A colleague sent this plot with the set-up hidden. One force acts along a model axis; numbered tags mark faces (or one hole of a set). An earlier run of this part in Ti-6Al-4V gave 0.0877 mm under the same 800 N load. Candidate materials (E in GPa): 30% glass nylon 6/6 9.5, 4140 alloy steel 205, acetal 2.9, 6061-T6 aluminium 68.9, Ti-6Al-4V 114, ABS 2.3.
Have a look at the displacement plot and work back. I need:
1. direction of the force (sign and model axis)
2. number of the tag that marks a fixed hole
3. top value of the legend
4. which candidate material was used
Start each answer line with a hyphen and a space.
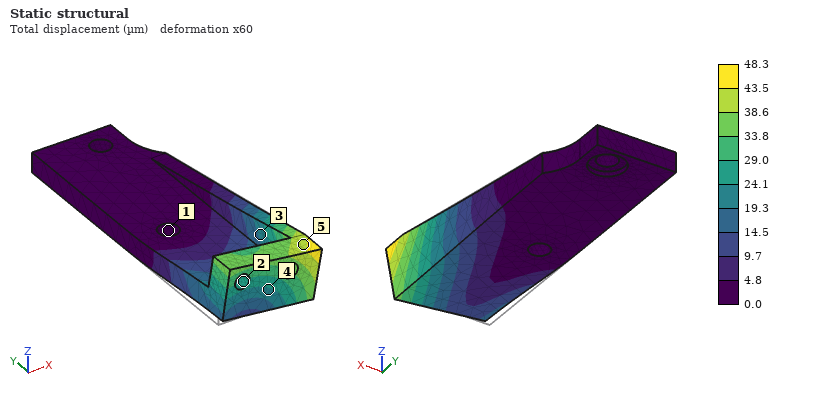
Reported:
- +X
- 1
- 48.3 µm
- 4140 alloy steel
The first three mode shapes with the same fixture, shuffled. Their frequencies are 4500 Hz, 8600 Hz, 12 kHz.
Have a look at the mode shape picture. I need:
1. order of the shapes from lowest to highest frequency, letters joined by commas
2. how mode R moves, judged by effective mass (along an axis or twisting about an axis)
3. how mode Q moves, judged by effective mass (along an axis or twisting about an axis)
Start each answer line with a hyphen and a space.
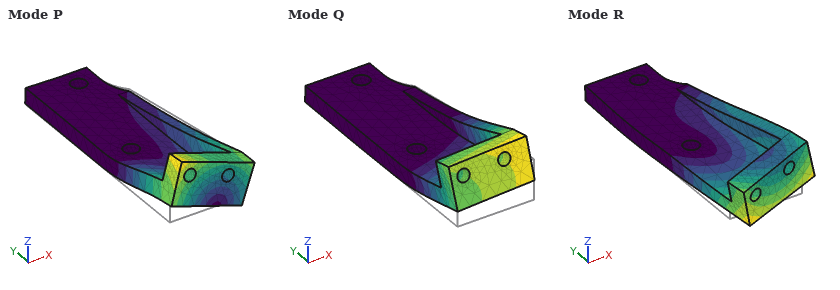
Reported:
- Q, P, R
- along X
- along Z
